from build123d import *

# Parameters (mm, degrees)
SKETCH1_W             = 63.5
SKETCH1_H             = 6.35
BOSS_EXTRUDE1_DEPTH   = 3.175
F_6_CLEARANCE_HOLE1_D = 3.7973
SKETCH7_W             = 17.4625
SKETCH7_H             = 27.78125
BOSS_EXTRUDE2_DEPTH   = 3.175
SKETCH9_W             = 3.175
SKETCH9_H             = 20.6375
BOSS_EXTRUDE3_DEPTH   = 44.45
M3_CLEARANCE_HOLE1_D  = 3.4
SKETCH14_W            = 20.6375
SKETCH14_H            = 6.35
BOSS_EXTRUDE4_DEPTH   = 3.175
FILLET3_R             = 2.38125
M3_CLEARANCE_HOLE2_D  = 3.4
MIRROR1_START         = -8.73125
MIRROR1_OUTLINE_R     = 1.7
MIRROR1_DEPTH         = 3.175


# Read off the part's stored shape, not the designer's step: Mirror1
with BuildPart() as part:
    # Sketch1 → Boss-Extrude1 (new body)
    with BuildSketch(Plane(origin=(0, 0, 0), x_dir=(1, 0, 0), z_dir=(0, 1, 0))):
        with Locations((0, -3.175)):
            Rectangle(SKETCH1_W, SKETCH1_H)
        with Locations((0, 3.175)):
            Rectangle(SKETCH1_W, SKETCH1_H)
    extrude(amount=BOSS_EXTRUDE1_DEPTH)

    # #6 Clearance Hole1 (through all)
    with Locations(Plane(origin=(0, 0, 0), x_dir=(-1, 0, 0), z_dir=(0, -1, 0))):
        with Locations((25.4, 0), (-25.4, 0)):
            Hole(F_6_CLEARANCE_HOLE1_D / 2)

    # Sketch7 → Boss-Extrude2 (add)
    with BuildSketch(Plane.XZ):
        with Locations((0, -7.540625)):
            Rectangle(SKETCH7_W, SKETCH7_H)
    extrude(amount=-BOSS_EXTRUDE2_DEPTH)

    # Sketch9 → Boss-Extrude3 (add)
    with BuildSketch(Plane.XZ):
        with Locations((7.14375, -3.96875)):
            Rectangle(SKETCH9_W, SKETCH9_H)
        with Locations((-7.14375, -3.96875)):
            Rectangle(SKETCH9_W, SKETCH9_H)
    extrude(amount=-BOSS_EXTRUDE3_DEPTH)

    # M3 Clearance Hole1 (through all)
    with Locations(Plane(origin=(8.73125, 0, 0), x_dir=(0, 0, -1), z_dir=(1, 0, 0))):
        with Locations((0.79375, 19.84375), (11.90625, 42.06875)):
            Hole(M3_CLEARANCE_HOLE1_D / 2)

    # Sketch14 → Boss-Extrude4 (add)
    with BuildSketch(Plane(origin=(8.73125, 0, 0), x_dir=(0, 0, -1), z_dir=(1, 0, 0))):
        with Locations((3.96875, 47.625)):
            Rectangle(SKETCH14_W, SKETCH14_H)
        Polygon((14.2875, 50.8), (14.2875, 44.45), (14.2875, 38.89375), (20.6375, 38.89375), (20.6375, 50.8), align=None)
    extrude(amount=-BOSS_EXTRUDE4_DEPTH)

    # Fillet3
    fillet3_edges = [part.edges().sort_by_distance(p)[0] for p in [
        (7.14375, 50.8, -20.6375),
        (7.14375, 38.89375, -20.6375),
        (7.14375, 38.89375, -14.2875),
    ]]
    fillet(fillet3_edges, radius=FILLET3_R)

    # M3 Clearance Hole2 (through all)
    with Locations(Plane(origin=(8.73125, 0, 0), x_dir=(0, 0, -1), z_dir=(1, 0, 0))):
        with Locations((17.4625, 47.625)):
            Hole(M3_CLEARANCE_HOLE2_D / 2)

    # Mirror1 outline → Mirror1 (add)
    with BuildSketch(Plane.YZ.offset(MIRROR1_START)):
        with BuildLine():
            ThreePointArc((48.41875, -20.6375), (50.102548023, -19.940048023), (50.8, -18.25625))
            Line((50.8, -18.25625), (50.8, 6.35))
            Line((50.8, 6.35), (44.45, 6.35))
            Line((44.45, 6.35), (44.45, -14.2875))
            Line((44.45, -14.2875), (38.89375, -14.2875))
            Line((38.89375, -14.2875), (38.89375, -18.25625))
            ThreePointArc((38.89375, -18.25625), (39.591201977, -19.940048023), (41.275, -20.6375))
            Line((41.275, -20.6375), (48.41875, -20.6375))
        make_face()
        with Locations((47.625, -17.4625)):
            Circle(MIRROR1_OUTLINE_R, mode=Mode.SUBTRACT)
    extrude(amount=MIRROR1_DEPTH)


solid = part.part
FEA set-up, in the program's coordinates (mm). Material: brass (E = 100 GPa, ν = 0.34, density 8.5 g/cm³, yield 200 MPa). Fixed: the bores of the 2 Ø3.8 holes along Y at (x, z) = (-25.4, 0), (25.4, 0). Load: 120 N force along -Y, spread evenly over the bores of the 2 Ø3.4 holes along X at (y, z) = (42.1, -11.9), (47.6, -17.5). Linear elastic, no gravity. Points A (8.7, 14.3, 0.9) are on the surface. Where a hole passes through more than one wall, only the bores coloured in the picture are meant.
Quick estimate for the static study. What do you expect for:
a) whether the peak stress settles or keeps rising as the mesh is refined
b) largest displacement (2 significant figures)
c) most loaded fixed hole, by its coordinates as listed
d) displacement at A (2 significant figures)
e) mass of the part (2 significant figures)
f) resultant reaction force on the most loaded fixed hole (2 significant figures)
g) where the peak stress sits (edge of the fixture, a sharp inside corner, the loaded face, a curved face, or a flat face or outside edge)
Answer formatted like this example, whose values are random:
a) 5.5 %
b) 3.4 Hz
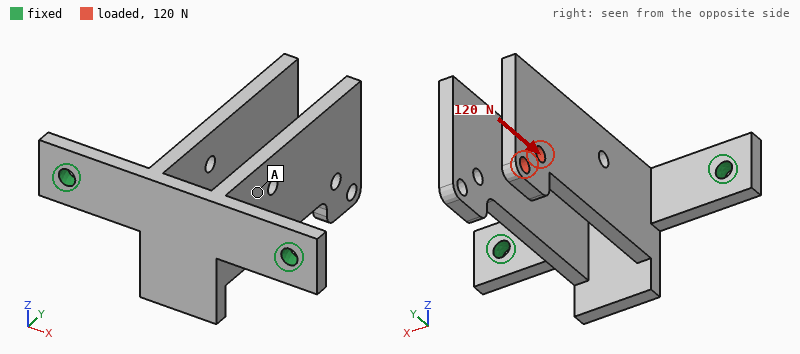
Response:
a) keeps rising
b) 0.18 mm
c) (-25.4, 0)
d) 0.035 mm
e) 84 g
f) 86 N
g) edge of the fixture
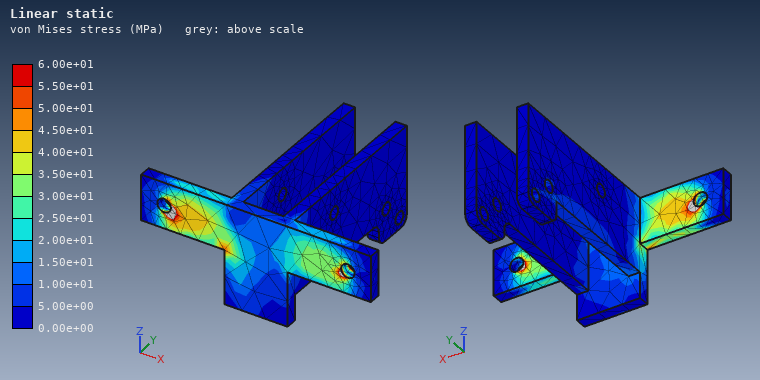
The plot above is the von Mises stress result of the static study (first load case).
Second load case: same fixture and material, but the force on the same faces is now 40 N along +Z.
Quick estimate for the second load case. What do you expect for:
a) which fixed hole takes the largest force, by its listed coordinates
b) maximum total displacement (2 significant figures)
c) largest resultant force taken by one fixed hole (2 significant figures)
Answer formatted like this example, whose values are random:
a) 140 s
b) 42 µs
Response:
a) (-25.4, 0)
b) 0.17 mm
c) 27 N
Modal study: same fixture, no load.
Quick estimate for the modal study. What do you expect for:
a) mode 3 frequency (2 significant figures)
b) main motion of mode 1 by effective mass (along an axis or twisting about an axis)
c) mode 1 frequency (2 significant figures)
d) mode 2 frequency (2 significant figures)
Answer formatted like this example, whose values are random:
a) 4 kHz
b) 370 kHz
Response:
a) 620 Hz
b) along Z
c) 520 Hz
d) 600 Hz
